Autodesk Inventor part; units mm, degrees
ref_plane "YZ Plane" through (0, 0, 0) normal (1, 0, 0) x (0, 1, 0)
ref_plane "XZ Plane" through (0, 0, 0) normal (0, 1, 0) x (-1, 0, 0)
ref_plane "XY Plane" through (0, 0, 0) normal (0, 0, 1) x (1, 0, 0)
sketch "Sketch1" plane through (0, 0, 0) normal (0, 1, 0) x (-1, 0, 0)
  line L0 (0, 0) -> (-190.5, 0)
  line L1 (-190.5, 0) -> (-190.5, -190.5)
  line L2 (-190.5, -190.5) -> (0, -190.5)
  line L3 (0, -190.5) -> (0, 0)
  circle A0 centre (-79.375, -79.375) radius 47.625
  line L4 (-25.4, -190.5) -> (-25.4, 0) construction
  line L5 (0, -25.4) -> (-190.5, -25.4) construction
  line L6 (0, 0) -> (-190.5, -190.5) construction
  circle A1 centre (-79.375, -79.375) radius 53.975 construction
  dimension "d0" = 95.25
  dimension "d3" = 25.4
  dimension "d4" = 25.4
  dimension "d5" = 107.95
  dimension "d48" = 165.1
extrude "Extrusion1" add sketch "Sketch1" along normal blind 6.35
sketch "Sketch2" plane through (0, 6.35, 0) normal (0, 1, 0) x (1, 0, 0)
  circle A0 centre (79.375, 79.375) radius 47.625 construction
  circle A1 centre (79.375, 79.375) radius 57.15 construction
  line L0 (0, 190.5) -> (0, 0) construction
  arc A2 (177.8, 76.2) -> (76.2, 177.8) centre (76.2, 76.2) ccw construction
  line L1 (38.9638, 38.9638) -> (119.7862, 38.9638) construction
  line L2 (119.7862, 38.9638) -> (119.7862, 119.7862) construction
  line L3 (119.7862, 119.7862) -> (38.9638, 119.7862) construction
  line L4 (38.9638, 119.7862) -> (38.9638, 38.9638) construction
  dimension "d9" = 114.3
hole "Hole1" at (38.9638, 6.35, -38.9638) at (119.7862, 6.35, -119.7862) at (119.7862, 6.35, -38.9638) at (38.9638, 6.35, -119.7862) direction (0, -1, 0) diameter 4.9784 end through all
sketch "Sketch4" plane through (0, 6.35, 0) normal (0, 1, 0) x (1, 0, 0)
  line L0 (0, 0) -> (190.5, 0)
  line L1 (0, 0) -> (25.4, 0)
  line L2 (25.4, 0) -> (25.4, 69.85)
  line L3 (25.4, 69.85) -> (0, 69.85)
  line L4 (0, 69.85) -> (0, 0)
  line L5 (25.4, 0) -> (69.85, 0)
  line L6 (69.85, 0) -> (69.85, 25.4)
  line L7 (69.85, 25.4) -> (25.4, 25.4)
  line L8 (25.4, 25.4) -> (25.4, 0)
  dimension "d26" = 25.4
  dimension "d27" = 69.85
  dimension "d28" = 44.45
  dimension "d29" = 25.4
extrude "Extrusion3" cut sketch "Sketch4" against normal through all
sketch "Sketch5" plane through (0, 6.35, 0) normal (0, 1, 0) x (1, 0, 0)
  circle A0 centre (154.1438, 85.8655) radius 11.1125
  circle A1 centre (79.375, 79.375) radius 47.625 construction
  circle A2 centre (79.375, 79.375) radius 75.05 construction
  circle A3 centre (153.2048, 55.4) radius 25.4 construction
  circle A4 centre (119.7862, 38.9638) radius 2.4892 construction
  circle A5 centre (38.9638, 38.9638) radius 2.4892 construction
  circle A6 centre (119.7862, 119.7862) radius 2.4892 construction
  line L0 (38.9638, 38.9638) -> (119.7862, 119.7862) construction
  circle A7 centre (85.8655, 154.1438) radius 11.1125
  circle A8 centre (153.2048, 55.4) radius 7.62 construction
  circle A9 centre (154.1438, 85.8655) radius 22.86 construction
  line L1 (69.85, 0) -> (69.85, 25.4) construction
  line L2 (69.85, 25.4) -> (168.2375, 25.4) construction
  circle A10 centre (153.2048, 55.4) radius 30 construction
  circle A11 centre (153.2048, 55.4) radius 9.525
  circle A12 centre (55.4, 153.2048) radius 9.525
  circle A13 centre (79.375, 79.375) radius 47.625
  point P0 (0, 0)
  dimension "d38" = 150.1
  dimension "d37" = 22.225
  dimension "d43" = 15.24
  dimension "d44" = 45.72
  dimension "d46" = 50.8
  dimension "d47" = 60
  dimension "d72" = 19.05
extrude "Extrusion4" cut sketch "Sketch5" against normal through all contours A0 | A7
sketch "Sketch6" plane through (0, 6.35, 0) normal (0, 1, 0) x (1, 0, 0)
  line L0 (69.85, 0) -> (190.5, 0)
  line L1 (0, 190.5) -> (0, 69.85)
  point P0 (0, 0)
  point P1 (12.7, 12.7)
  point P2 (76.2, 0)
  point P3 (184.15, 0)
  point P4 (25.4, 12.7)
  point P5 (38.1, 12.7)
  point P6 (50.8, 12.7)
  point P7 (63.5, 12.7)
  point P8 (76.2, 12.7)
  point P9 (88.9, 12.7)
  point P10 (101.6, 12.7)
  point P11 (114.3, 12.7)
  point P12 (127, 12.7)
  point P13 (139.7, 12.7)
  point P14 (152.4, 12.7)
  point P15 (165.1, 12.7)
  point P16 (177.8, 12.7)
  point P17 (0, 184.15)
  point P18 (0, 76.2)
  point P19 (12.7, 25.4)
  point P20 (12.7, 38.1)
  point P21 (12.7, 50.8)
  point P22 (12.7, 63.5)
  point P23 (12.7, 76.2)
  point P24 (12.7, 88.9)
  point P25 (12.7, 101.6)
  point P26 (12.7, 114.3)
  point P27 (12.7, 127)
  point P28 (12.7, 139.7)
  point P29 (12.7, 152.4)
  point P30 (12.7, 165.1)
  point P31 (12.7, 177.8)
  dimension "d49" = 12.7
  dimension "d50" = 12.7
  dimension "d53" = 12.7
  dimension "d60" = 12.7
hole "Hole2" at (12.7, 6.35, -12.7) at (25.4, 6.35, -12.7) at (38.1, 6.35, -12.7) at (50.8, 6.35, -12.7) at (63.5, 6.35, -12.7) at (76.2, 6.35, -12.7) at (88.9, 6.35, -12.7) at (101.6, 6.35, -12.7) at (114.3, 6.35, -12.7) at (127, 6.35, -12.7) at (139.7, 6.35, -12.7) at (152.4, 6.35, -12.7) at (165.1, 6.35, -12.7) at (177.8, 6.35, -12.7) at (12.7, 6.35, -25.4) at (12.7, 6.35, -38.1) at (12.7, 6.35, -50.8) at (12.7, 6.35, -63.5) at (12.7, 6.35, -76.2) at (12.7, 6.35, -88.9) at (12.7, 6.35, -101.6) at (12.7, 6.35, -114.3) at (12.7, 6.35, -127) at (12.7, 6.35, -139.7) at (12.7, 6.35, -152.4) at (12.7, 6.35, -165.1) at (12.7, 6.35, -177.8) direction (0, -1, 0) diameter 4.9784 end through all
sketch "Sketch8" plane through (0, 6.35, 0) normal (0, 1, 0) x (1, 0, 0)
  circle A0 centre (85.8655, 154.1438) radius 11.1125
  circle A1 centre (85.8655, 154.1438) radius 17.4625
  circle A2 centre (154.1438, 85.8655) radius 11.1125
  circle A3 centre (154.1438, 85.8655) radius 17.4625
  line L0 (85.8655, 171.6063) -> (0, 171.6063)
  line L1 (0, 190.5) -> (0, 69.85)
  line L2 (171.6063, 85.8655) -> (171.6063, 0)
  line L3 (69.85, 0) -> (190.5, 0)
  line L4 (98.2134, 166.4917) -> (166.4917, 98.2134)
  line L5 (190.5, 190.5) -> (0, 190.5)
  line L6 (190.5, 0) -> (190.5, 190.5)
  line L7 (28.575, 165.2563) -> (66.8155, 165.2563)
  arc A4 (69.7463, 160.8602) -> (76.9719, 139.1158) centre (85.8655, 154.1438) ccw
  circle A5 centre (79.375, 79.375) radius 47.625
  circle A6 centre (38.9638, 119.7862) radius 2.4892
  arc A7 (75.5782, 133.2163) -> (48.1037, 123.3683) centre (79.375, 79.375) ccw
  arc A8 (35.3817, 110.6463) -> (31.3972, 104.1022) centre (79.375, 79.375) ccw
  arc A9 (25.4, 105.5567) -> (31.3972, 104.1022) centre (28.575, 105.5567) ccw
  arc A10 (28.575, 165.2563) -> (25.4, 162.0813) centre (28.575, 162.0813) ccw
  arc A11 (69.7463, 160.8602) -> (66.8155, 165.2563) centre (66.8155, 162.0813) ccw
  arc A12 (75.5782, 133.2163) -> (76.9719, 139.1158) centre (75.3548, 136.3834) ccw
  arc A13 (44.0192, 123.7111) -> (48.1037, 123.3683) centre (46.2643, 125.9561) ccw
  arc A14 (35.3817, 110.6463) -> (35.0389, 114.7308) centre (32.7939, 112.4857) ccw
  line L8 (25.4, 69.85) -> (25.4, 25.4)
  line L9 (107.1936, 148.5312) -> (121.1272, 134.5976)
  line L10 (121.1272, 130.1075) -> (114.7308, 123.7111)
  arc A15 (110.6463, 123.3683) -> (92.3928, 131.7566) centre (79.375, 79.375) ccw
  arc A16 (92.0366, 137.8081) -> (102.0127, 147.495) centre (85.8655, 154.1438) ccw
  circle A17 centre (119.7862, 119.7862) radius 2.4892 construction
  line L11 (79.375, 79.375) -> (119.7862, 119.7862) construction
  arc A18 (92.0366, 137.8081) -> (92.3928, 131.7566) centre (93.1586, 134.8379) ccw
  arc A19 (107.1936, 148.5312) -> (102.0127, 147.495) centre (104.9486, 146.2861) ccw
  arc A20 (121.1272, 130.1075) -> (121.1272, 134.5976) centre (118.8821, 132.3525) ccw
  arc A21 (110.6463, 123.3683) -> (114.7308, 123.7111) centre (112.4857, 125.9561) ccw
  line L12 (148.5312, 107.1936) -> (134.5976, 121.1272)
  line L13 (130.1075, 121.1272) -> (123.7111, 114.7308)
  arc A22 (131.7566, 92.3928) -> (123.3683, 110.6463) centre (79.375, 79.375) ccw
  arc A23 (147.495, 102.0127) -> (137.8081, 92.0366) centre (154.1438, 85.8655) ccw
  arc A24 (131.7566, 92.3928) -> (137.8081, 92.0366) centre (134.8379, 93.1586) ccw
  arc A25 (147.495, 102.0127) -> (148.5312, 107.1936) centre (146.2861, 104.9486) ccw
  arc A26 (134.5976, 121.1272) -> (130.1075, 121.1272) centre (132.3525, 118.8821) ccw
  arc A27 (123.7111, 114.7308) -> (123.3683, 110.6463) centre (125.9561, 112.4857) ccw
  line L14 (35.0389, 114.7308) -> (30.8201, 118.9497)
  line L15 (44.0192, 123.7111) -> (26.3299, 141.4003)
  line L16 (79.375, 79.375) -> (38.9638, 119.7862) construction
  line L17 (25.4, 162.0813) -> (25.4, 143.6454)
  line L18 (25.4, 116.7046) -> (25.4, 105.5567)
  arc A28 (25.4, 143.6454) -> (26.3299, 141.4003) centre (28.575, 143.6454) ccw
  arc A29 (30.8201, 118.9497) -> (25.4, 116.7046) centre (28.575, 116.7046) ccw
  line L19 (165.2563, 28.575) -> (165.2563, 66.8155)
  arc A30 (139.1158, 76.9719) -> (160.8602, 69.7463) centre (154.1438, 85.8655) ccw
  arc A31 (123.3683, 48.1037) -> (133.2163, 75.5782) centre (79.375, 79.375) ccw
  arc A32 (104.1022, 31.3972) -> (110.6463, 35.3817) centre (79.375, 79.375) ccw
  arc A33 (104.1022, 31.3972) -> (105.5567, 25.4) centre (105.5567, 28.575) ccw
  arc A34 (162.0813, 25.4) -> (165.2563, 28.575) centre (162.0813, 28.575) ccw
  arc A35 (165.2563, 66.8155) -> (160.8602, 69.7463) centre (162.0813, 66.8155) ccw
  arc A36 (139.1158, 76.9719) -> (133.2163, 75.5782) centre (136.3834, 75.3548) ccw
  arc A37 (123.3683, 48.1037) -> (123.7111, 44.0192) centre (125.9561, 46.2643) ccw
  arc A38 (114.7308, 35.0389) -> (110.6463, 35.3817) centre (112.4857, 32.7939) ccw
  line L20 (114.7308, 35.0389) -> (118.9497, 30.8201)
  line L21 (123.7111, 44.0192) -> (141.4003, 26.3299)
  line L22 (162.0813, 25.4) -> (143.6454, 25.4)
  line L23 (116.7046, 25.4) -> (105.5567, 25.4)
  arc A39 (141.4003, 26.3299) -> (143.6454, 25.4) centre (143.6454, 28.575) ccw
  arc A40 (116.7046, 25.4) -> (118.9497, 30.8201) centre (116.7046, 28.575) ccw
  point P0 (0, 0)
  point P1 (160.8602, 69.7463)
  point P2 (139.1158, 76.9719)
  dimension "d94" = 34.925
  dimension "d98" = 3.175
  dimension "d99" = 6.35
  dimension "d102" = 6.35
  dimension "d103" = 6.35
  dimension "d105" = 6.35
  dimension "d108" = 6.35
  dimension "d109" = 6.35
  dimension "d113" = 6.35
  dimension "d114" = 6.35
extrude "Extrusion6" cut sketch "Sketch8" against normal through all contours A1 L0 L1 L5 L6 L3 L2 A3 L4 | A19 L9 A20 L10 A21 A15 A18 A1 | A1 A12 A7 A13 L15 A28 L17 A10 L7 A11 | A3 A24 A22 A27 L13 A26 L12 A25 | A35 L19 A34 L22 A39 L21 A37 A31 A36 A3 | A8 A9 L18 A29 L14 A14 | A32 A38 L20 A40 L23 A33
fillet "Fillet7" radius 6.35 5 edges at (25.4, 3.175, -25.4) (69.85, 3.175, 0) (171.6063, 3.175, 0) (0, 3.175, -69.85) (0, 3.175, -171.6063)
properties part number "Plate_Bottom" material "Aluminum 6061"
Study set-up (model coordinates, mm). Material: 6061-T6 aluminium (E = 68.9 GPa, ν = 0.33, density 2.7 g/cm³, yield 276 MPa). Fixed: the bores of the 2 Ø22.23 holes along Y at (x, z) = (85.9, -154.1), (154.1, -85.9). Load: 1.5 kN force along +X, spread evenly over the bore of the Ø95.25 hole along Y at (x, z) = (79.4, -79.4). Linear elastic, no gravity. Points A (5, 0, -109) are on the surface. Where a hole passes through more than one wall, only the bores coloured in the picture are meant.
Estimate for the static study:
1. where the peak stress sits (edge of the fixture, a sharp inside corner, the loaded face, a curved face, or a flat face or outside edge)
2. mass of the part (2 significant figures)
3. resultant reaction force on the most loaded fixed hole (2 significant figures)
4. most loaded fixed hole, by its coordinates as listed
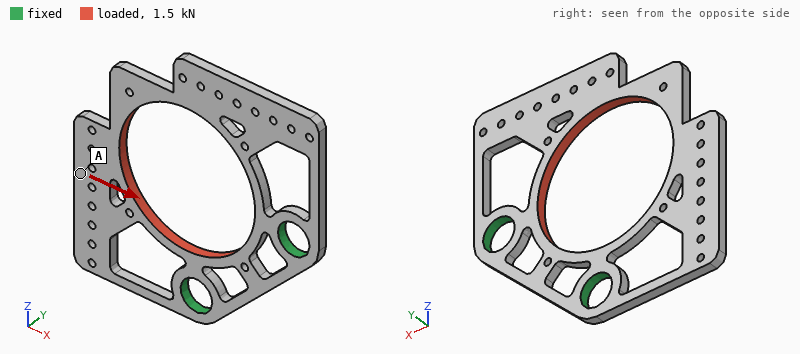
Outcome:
a curved face
180 g
840 N
(154.1, -85.9)
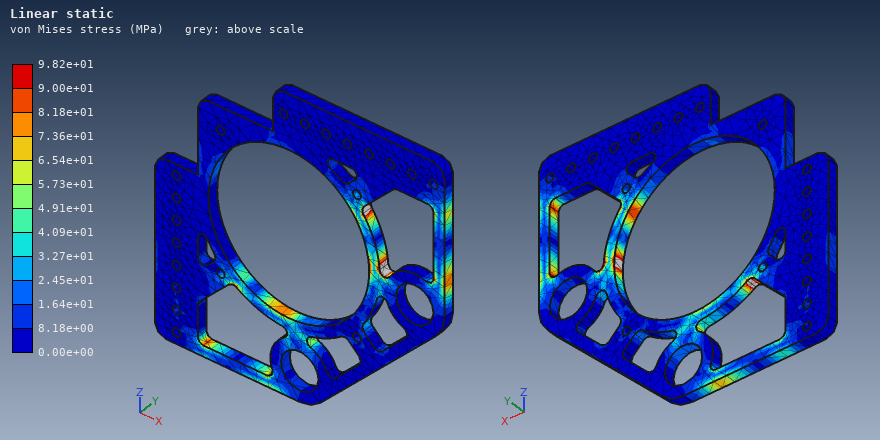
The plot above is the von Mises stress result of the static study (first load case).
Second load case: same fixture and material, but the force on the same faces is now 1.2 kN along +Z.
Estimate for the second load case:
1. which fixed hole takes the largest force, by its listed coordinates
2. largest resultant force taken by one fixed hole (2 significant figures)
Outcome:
(85.9, -154.1)
670 N
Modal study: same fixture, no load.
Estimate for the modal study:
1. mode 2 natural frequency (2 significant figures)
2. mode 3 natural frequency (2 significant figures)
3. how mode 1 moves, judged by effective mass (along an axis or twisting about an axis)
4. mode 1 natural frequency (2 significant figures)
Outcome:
370 Hz
700 Hz
along Y
210 Hz
